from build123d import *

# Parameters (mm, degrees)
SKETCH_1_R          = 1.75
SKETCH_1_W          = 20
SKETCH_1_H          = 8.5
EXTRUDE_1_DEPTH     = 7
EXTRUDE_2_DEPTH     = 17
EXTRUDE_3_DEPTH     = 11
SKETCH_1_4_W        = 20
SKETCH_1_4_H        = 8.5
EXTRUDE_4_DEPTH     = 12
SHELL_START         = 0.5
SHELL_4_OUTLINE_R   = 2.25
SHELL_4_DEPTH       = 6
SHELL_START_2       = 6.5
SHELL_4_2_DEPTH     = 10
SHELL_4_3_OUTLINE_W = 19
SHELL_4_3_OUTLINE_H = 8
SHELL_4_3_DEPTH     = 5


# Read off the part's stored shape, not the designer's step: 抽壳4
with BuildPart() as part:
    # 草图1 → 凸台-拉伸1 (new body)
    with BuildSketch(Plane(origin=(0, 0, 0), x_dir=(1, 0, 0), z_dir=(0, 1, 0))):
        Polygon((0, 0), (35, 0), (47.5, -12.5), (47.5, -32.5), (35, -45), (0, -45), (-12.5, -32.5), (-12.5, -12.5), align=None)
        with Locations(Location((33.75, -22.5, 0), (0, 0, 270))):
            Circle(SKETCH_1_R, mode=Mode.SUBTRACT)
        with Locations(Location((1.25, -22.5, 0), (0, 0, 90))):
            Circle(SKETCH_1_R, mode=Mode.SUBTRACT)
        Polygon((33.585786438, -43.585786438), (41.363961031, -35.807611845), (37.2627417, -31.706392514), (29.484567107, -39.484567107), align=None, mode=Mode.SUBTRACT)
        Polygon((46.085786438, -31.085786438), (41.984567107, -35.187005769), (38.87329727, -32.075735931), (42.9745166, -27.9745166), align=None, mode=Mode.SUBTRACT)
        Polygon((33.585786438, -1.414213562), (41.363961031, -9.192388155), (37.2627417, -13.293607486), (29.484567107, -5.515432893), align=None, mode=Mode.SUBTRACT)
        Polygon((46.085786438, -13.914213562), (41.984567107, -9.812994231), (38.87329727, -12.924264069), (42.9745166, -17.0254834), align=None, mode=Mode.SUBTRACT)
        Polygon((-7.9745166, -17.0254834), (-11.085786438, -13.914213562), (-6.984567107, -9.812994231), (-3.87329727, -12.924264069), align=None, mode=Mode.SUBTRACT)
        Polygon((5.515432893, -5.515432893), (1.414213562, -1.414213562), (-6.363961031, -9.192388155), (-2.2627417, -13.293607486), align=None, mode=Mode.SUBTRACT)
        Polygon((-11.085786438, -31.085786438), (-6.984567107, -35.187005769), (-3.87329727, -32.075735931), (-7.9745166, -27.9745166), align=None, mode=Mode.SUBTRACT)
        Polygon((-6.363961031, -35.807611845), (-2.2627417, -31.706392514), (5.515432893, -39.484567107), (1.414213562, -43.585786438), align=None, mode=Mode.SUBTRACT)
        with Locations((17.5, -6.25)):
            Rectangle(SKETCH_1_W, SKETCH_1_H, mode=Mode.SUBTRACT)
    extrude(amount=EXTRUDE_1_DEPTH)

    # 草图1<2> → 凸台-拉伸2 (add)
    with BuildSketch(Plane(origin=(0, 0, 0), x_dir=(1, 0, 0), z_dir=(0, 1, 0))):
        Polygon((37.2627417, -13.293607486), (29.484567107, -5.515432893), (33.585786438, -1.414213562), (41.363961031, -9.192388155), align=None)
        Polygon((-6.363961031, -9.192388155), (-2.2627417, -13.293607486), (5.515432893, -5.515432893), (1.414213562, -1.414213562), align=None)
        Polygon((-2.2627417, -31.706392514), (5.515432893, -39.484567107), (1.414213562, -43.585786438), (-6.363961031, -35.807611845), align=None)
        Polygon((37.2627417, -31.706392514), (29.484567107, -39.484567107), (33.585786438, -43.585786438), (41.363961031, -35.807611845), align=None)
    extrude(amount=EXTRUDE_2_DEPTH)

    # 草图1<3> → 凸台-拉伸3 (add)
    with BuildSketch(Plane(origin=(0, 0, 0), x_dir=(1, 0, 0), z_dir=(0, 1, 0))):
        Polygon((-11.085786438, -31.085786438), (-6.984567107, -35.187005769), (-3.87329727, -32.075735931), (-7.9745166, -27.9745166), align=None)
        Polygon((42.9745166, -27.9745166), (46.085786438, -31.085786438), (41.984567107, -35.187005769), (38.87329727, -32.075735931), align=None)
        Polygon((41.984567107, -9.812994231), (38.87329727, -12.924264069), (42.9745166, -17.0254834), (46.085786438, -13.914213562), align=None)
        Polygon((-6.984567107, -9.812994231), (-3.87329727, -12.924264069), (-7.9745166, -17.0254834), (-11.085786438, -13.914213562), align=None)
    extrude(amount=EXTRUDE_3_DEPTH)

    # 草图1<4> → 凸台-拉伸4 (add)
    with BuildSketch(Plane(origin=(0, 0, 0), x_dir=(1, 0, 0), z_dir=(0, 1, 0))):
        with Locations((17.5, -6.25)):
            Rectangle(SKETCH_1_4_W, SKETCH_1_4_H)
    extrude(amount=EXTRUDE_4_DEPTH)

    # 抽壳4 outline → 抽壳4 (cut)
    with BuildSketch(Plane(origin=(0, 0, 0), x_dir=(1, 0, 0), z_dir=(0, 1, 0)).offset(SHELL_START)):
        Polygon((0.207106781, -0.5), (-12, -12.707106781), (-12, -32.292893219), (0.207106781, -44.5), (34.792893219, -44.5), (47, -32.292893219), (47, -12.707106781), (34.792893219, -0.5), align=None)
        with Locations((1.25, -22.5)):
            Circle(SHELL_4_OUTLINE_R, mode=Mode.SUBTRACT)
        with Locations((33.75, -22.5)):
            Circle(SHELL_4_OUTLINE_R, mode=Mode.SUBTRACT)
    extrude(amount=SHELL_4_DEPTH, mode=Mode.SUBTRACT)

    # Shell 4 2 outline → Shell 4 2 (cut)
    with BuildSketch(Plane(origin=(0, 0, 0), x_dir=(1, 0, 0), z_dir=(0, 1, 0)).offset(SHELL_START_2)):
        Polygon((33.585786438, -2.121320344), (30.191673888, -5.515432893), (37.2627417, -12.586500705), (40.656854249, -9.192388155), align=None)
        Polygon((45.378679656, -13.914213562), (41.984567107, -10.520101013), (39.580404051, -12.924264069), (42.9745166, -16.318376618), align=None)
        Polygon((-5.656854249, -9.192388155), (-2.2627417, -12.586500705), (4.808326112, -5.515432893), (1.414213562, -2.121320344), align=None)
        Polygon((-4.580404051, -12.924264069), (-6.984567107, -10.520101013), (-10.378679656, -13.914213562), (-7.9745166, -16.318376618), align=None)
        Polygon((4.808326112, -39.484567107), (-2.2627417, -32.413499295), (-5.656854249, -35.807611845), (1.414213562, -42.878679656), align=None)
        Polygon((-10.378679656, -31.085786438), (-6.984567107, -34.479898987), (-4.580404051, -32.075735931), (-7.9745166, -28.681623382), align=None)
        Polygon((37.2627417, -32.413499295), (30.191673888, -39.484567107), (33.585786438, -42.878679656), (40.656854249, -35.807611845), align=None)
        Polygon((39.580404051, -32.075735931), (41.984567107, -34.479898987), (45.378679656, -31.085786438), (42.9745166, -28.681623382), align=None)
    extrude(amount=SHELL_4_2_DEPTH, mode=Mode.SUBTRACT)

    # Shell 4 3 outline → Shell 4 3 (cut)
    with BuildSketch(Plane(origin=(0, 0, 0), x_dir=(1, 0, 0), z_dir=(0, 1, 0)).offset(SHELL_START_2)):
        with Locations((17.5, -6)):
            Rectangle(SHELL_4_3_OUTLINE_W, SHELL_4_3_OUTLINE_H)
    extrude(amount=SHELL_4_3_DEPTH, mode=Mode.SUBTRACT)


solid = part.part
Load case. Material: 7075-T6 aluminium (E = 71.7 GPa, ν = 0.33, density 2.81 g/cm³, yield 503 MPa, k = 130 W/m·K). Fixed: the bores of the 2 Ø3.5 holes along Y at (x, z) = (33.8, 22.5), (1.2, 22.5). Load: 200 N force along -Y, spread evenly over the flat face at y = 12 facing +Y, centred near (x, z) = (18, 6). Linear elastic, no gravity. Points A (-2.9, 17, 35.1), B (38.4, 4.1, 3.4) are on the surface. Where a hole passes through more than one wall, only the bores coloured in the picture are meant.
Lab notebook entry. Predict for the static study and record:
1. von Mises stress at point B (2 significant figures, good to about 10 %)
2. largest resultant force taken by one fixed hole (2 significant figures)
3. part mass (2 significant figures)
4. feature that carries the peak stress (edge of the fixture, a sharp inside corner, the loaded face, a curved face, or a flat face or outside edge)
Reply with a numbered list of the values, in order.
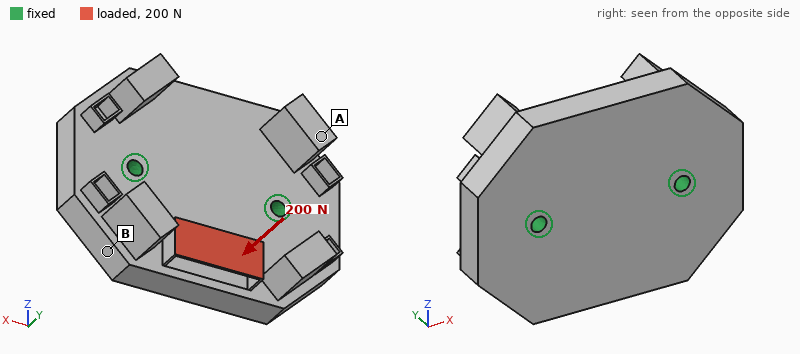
1. 55 MPa
2. 100 N
3. 11 g
4. a flat face or outside edge
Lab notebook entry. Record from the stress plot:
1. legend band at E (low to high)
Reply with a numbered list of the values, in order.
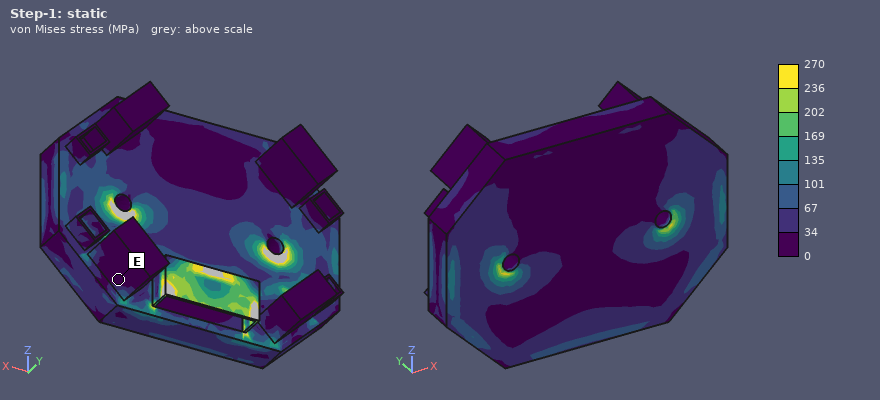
1. 0 to 34 MPa
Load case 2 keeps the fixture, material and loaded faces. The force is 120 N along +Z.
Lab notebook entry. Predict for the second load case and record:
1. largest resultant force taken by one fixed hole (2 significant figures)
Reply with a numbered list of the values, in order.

1. 65 N
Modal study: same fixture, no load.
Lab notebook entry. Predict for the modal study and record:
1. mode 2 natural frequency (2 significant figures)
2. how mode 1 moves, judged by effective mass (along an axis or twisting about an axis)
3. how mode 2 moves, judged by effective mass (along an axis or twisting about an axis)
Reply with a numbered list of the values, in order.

1. 2400 Hz
2. along Y
3. twisting about X
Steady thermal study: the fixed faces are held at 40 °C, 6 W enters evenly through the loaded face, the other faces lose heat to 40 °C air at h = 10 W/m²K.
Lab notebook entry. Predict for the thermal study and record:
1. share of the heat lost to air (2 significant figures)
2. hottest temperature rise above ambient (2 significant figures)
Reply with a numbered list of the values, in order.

1. 17 %
2. 49 K
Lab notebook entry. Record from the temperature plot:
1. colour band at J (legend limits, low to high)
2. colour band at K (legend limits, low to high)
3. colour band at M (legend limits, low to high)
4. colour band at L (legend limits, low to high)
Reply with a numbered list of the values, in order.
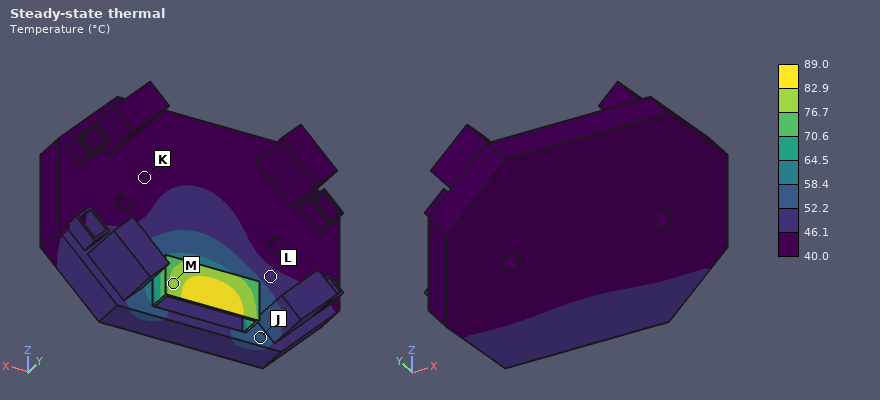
1. 52.2 to 58.4 °C
2. 40.0 to 46.1 °C
3. 76.7 to 82.9 °C
4. 46.1 to 52.2 °C
